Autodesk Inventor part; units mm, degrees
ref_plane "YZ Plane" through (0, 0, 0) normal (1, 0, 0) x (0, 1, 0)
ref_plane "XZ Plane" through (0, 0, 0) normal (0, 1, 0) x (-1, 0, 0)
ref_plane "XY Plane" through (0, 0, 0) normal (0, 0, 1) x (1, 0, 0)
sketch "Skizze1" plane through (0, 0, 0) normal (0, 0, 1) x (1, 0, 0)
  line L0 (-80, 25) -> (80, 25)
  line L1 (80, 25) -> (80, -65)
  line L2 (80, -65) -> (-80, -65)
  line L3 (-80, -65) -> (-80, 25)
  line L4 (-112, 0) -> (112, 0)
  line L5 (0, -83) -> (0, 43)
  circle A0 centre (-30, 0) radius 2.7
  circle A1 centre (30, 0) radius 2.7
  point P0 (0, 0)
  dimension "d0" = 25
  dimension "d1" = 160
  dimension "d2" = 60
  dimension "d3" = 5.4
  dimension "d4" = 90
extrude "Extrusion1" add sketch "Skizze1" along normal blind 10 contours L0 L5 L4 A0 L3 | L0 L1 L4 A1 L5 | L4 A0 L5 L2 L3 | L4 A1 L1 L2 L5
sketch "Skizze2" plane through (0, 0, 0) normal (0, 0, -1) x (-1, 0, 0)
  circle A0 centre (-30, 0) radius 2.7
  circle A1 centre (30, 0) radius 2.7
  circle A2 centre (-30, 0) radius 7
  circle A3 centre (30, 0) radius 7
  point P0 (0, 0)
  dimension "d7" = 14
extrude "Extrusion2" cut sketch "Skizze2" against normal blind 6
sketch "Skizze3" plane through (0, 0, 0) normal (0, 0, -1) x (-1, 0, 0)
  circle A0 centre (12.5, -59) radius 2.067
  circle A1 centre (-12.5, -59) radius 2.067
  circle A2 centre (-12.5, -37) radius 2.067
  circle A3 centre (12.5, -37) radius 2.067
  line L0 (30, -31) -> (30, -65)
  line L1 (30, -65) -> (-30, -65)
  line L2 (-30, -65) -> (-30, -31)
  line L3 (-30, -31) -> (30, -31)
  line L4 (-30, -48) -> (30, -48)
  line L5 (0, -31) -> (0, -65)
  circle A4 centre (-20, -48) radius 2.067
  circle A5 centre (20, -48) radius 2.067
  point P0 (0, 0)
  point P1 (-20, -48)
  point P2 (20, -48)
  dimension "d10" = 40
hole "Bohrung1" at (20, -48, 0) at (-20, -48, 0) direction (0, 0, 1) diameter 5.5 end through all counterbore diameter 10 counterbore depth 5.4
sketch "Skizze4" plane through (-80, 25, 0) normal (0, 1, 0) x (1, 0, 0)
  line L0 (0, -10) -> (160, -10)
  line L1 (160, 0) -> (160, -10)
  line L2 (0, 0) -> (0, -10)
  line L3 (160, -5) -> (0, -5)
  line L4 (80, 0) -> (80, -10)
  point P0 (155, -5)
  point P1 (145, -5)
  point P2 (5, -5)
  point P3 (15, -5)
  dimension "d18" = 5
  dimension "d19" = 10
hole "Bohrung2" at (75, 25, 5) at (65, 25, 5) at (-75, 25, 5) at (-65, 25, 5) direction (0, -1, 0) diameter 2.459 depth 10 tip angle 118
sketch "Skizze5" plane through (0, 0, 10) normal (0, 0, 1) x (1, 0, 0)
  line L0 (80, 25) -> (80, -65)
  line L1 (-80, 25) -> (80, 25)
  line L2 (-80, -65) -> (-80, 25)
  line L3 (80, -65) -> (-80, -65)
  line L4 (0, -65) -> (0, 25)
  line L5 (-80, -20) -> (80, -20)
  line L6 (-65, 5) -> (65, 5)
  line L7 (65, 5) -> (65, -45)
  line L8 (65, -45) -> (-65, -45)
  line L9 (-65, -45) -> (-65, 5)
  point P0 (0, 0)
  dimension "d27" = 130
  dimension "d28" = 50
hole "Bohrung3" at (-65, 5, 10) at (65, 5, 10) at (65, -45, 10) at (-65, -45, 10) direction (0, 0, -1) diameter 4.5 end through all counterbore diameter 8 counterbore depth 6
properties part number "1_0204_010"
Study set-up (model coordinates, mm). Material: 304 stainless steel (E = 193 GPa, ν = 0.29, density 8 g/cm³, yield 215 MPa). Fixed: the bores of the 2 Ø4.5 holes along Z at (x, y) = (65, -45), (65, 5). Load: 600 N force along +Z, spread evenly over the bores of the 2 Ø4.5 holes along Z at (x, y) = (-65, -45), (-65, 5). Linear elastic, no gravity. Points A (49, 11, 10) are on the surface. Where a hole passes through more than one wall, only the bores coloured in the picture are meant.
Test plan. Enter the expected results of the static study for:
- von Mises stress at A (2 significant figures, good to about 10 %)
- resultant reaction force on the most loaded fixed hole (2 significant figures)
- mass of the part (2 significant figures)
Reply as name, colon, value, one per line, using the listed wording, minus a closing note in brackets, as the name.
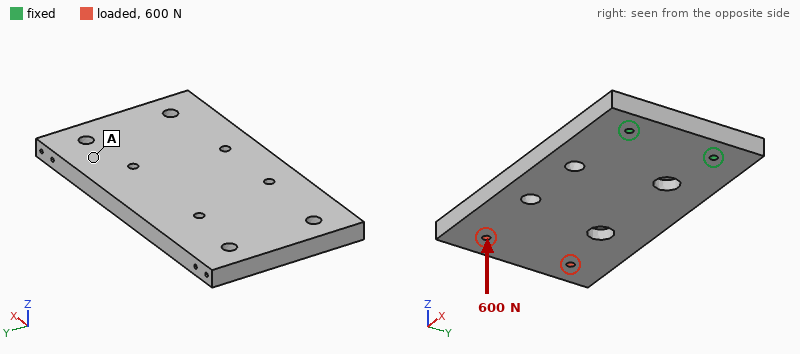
von Mises stress at A: 44 MPa
resultant reaction force on the most loaded fixed hole: 570 N
mass of the part: 1.1 kg
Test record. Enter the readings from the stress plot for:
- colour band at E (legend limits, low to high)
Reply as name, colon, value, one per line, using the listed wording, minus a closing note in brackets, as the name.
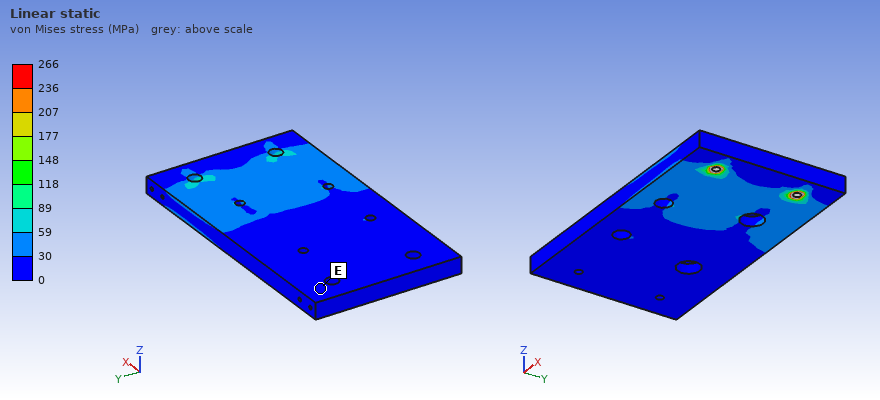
colour band at E: 0 to 30 MPa
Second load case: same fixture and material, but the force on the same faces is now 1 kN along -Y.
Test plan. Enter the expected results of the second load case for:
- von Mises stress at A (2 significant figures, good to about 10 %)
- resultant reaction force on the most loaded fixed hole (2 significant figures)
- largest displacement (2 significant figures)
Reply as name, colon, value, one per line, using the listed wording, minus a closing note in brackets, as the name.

von Mises stress at A: 6.7 MPa
resultant reaction force on the most loaded fixed hole: 2.6 kN
largest displacement: 27 µm
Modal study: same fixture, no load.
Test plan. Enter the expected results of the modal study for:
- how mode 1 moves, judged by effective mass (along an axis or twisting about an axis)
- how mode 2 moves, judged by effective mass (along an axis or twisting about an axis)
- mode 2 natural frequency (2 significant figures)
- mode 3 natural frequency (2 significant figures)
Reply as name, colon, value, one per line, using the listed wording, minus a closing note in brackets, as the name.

how mode 1 moves, judged by effective mass: along Z
how mode 2 moves, judged by effective mass: twisting about X
mode 2 natural frequency: 1200 Hz
mode 3 natural frequency: 1800 Hz
